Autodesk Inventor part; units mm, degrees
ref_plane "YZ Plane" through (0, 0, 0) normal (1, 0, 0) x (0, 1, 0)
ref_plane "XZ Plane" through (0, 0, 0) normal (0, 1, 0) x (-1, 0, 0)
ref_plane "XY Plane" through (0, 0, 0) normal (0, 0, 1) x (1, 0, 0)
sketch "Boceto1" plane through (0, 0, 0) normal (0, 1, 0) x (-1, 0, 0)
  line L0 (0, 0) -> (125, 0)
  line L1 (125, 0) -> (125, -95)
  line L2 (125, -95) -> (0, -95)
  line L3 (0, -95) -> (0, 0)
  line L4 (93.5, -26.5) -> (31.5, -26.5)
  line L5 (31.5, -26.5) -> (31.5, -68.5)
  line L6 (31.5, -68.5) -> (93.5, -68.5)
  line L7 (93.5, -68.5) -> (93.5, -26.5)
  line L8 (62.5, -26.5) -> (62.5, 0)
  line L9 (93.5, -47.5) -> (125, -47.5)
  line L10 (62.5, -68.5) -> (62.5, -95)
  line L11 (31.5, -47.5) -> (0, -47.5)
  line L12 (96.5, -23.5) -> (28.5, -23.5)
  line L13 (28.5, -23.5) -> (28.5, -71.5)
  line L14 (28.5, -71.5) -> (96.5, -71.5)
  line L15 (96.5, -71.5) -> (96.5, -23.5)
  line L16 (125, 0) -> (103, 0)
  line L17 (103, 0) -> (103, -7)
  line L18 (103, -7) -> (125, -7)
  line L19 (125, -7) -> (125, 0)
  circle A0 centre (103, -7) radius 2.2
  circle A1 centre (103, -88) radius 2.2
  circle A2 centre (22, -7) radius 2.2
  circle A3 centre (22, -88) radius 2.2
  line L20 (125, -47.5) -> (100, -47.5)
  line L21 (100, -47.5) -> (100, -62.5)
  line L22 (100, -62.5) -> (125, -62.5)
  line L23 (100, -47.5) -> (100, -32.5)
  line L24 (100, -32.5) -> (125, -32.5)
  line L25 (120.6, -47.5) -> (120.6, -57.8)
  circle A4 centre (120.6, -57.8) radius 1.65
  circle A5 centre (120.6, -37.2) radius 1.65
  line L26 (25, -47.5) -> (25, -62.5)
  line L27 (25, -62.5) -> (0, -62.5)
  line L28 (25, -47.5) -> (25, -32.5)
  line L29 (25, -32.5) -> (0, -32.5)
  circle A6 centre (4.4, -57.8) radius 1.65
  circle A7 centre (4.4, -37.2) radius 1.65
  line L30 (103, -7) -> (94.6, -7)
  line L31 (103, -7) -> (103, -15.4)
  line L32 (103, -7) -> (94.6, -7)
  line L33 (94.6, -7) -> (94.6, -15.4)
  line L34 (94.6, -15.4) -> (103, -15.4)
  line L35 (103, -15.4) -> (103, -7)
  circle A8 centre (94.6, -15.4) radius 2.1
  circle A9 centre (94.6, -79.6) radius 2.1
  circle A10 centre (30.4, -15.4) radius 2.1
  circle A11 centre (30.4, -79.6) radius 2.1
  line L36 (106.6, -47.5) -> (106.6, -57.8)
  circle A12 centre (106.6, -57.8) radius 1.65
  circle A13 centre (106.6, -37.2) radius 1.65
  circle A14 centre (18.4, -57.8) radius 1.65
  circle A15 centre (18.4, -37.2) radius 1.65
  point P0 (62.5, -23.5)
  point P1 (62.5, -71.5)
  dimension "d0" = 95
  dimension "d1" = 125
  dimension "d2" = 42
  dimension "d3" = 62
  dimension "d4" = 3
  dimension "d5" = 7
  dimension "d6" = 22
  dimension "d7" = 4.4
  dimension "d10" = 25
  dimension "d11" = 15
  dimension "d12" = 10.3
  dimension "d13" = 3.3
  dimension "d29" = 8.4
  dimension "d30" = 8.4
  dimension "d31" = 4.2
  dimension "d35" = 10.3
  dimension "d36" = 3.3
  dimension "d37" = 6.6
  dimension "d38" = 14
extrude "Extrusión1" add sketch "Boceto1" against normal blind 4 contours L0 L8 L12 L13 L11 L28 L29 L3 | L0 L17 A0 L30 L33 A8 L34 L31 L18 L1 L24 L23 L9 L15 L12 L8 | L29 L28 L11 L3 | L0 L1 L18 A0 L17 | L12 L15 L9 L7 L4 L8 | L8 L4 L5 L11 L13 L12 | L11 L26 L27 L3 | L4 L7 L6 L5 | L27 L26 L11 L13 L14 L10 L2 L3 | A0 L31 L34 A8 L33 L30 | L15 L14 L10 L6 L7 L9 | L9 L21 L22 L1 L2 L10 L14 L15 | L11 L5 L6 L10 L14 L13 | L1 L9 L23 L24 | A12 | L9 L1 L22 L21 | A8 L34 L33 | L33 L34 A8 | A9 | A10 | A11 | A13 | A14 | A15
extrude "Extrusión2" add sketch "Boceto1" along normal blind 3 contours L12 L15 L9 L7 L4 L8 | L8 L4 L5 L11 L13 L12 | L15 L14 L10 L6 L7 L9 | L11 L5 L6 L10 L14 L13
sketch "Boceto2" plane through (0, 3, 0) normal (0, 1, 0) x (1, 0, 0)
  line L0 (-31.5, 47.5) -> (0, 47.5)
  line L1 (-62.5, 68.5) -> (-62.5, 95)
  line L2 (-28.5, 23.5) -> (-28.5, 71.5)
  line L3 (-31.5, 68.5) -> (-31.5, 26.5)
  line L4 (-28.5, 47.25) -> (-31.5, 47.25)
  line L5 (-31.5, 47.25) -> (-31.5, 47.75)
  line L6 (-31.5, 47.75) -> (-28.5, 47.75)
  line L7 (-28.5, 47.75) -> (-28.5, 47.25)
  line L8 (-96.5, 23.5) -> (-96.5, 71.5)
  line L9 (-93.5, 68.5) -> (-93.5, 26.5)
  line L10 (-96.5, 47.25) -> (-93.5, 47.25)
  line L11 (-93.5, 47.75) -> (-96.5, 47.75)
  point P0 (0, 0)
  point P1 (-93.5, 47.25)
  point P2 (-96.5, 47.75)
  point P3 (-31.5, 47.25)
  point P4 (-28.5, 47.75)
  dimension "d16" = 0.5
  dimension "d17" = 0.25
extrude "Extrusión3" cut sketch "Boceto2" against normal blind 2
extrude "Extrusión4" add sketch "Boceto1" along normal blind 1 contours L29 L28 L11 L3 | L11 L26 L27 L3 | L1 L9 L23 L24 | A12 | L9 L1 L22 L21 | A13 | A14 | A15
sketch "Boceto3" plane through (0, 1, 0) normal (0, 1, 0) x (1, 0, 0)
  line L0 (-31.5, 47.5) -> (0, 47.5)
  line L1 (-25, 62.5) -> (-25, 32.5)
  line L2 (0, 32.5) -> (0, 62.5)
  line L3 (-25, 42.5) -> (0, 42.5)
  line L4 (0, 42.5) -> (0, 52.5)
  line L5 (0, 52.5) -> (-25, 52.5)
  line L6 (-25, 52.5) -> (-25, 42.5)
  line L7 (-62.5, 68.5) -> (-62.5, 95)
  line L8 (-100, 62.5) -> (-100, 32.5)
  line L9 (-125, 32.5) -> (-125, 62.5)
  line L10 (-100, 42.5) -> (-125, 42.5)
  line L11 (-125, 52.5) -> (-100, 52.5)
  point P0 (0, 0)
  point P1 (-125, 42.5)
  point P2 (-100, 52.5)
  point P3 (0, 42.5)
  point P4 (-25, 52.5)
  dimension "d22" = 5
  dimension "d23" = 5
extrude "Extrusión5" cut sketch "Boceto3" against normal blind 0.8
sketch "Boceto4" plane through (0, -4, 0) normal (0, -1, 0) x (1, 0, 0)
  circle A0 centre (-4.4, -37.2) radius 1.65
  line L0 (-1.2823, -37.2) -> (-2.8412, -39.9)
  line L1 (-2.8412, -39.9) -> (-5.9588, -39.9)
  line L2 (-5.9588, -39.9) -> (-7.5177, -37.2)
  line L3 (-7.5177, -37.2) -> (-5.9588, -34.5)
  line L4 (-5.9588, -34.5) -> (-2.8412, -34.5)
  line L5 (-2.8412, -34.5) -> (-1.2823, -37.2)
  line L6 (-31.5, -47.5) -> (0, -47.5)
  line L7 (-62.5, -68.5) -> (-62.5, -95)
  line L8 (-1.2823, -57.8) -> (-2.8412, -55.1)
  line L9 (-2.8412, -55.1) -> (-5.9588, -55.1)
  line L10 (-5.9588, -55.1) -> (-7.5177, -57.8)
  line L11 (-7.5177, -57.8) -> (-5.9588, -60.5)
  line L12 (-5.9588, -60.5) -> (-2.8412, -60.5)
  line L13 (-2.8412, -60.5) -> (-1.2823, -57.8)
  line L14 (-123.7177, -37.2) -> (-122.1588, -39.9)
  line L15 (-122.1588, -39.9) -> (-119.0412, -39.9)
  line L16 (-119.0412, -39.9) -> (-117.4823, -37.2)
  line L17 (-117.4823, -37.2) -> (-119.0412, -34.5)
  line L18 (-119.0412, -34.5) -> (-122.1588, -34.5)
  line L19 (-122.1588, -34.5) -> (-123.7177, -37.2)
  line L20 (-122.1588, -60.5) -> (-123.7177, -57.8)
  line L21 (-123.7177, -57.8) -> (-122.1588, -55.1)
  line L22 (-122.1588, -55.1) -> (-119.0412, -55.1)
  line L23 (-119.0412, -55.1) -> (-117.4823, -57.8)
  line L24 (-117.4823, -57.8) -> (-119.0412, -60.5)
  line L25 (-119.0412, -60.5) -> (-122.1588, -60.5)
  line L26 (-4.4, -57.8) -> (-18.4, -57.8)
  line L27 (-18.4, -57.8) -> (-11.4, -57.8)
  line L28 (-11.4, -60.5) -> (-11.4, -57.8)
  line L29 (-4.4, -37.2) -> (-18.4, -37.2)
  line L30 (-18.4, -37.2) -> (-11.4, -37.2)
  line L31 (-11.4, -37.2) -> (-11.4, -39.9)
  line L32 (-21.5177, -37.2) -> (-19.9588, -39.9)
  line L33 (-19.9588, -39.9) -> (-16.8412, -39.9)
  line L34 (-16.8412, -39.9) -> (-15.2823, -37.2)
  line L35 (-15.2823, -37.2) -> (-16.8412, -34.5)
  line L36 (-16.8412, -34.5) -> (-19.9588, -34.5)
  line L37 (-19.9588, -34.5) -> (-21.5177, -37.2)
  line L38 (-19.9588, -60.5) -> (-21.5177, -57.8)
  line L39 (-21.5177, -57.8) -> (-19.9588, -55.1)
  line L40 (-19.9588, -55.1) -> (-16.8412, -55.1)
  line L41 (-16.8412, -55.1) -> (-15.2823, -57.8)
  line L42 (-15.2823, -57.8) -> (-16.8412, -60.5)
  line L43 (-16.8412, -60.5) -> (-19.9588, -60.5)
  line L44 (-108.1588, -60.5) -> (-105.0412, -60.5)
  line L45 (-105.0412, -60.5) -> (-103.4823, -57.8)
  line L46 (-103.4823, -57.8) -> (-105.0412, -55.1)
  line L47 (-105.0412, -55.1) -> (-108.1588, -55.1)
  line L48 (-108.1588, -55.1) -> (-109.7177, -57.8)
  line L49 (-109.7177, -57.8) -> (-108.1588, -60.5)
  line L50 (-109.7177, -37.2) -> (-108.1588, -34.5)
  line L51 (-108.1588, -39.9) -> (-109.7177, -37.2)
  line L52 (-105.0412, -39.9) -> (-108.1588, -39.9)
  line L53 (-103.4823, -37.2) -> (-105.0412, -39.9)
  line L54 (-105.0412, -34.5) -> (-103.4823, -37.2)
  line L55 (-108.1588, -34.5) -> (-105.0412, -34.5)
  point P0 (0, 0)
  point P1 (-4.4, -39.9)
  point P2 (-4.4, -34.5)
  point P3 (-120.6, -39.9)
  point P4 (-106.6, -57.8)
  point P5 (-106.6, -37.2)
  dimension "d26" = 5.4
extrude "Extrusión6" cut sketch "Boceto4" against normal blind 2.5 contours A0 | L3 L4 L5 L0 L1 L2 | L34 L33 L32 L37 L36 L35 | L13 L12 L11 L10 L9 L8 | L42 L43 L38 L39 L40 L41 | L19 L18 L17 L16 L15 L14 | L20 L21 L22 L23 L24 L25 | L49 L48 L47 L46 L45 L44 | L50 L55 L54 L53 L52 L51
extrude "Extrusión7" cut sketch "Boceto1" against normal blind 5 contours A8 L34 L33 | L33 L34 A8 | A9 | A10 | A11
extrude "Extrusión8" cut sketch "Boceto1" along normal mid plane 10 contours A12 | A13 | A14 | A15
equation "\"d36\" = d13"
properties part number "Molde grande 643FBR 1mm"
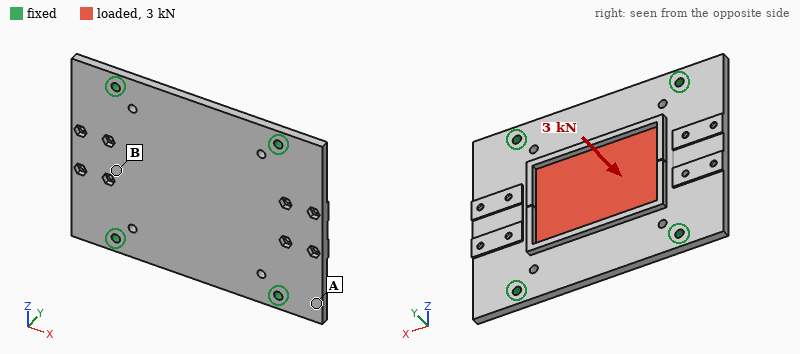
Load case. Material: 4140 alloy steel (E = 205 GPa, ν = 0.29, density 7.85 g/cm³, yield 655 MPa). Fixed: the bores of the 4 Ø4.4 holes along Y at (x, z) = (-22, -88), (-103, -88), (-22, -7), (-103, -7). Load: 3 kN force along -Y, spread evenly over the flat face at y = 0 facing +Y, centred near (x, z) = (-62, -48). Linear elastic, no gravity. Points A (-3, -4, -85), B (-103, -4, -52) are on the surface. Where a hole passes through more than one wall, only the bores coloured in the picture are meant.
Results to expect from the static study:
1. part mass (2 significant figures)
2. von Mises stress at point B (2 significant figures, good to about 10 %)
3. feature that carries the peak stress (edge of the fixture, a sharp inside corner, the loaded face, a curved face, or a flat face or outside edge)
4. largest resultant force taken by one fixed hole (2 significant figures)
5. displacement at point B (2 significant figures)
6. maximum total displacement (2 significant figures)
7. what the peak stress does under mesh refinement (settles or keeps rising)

390 g
51 MPa
edge of the fixture
820 N
0.058 mm
0.14 mm
keeps rising
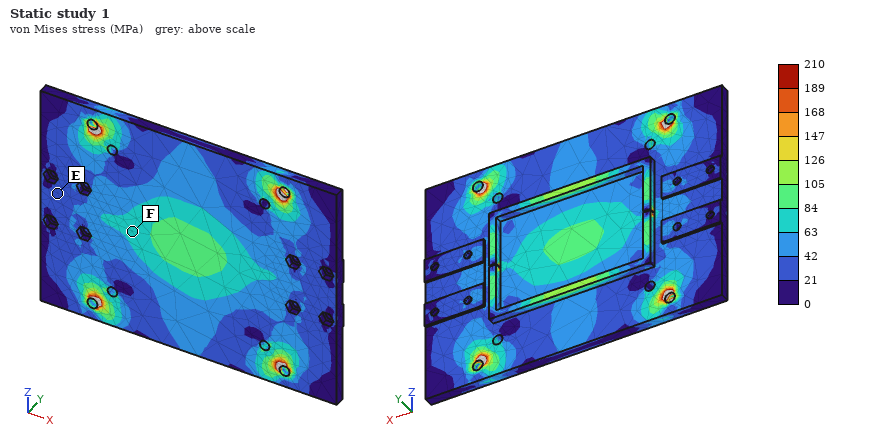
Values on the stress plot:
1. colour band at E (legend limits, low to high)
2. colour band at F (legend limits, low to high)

21 to 42 MPa
63 to 84 MPa
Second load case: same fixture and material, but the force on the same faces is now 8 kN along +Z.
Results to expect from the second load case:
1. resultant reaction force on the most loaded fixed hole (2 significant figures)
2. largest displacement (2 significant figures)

2.2 kN
11 µm
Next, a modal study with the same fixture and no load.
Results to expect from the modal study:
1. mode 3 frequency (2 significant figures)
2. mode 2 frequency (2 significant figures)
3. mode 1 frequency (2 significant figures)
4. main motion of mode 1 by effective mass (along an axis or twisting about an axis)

3000 Hz
2900 Hz
2200 Hz
along Y
